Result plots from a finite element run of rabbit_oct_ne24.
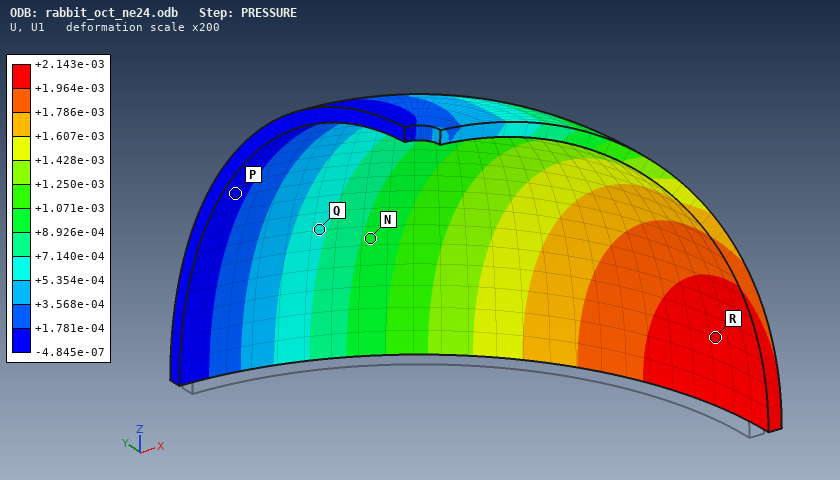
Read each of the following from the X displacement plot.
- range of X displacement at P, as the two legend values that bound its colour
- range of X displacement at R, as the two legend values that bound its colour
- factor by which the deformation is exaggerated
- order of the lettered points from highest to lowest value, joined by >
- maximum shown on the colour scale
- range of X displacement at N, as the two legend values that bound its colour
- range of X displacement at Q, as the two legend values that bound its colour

-4.845e-07 to +1.781e-04
+1.964e-03 to +2.143e-03
200
R > N > Q > P
+2.143e-03
+8.926e-04 to +1.071e-03
+5.354e-04 to +7.140e-04
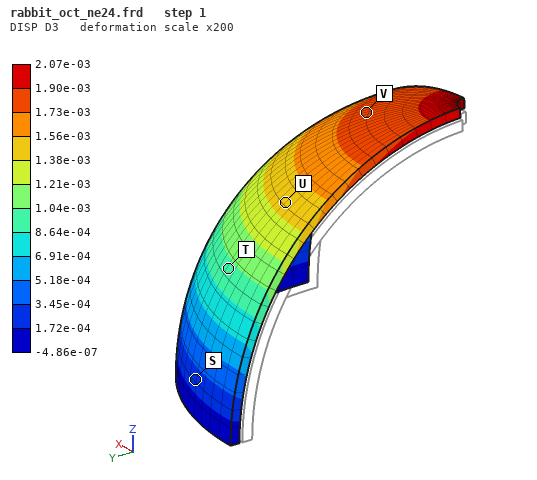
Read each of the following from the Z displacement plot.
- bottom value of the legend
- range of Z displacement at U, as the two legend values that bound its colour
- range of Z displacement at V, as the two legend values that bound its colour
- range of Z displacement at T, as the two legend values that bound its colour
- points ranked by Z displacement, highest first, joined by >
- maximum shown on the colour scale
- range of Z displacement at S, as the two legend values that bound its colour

-4.86e-07
1.38e-03 to 1.56e-03
1.73e-03 to 1.90e-03
8.64e-04 to 1.04e-03
V > U > T > S
2.07e-03
1.72e-04 to 3.45e-04
